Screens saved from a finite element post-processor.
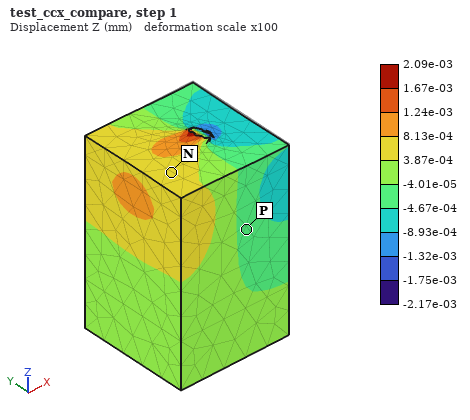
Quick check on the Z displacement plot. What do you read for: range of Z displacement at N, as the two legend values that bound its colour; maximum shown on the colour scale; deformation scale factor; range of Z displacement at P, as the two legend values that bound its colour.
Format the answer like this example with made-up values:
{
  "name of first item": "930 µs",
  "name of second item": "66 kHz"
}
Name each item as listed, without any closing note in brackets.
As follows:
{
  "range of Z displacement at N, as the two legend values that bound its colour": "3.87e-04 to 8.13e-04 mm",
  "maximum shown on the colour scale": "2.09e-03 mm",
  "deformation scale factor": "100",
  "range of Z displacement at P, as the two legend values that bound its colour": "-4.67e-04 to -4.01e-05 mm"
}
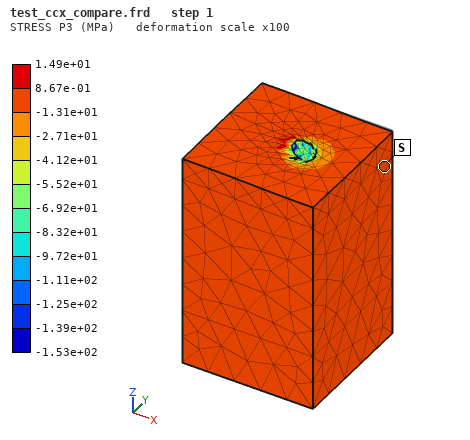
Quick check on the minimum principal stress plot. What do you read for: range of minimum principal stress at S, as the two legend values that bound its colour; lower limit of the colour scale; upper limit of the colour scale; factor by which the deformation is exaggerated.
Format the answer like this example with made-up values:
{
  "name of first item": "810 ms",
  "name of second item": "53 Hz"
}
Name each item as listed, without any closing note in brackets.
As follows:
{
  "range of minimum principal stress at S, as the two legend values that bound its colour": "-1.31e+01 to 8.67e-01 MPa",
  "lower limit of the colour scale": "-1.53e+02 MPa",
  "upper limit of the colour scale": "1.49e+01 MPa",
  "factor by which the deformation is exaggerated": "100"
}
